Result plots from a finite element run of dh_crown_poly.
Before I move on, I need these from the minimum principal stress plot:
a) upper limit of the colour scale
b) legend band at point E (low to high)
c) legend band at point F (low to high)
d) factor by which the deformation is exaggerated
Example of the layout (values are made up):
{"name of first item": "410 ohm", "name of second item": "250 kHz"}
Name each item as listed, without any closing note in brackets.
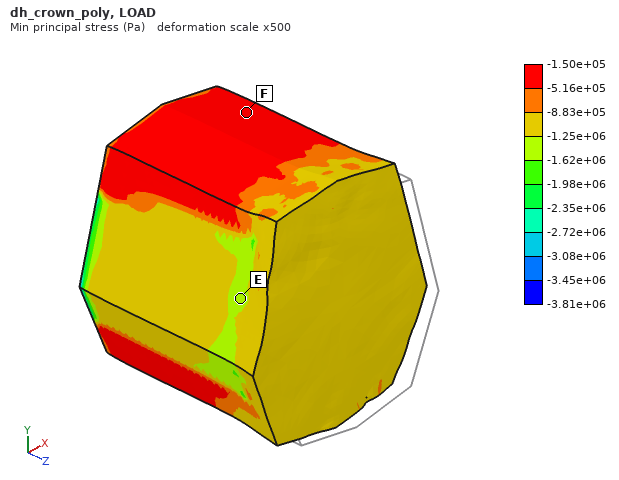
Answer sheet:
{"upper limit of the colour scale": "-1.50e+05 Pa", "legend band at point E": "-1.62e+06 to -1.25e+06 Pa", "legend band at point F": "-5.16e+05 to -1.50e+05 Pa", "factor by which the deformation is exaggerated": "500"}
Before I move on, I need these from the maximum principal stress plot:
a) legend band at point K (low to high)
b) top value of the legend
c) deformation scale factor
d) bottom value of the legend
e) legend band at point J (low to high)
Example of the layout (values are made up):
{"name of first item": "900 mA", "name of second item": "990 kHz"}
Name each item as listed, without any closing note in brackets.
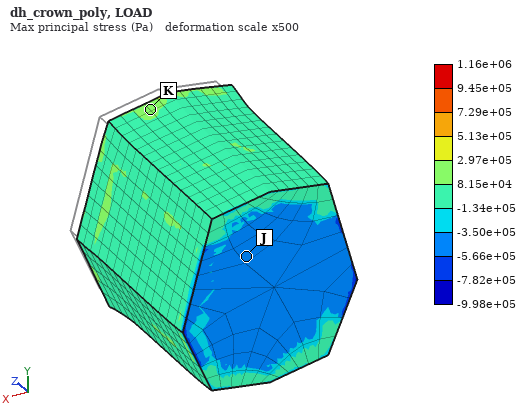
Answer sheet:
{"legend band at point K": "8.15e+04 to 2.97e+05 Pa", "top value of the legend": "1.16e+06 Pa", "deformation scale factor": "500", "bottom value of the legend": "-9.98e+05 Pa", "legend band at point J": "-5.66e+05 to -3.50e+05 Pa"}
